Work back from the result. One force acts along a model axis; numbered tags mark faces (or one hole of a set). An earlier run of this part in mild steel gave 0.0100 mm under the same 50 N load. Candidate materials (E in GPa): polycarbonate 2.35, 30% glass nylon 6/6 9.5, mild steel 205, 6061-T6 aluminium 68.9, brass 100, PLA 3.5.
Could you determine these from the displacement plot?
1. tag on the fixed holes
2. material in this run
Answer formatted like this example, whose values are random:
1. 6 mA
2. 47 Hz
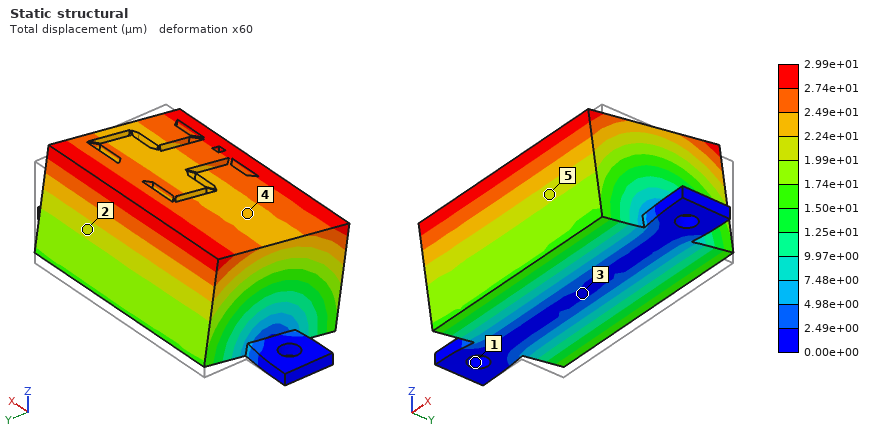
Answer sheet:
1. 1
2. 6061-T6 aluminium
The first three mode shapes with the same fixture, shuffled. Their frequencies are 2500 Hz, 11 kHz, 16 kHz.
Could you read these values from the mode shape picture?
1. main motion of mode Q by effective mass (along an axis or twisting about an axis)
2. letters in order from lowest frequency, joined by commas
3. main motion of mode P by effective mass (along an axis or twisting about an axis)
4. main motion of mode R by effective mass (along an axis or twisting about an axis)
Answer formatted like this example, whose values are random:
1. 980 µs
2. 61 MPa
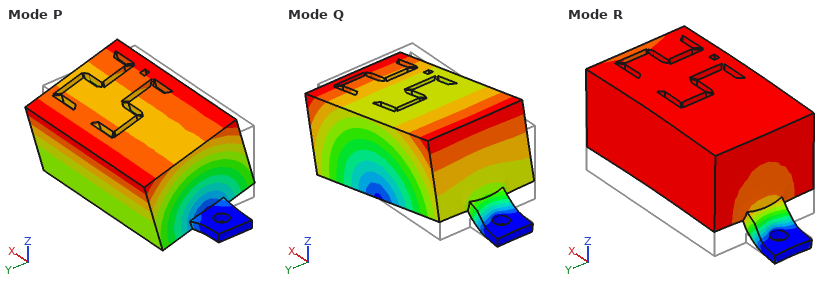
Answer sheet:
1. along X
2. P, R, Q
3. along Y
4. along Z
